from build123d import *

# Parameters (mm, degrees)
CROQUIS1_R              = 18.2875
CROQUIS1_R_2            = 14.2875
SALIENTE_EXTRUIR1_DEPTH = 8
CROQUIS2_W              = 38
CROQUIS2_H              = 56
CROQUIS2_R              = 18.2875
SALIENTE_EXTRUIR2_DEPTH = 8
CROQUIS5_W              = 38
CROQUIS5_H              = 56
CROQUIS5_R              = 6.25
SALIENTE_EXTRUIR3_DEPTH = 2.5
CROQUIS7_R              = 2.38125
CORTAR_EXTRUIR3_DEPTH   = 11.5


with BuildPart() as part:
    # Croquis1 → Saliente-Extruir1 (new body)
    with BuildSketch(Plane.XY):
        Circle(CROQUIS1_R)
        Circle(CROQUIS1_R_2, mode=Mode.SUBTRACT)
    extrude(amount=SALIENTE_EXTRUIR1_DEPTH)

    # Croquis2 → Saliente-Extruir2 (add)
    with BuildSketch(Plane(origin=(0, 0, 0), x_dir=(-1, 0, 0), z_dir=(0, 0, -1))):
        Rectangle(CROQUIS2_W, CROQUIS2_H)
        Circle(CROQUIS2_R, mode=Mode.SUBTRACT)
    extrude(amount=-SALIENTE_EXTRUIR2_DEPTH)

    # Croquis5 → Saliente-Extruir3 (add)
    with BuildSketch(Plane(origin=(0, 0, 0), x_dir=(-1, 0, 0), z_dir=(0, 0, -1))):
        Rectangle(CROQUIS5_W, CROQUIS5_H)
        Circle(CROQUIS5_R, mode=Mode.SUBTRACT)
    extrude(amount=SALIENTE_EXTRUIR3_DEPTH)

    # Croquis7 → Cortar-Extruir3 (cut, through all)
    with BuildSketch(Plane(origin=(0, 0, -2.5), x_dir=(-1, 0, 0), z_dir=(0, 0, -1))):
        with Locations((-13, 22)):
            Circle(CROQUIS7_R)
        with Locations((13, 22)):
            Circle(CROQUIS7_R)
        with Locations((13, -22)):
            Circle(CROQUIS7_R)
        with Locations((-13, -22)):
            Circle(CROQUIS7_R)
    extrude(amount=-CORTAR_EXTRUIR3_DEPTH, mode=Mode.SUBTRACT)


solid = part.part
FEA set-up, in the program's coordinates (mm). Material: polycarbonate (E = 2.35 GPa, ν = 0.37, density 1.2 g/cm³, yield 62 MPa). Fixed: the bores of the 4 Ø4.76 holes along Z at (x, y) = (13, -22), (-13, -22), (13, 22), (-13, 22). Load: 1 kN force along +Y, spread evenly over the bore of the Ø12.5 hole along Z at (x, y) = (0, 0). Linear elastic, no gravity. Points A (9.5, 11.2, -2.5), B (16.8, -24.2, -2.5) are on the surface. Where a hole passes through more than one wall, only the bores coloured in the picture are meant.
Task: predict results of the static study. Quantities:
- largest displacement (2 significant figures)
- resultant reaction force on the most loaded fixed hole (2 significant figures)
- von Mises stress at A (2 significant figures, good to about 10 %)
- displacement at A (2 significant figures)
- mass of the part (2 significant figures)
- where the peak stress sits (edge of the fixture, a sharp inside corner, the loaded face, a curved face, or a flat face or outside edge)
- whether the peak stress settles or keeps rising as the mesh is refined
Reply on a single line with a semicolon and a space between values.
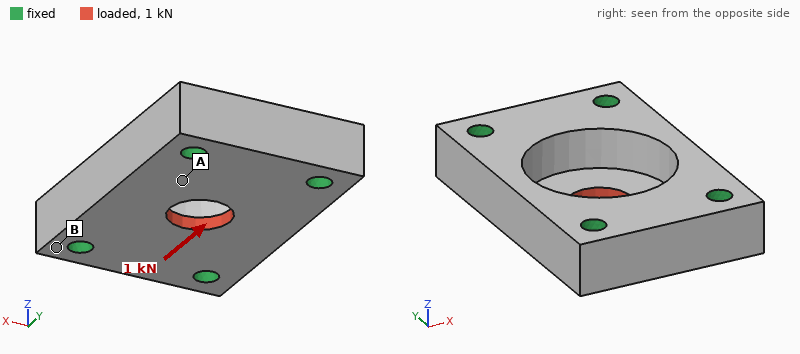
65 µm; 260 N; 6.0 MPa; 25 µm; 19 g; a sharp inside corner; keeps rising
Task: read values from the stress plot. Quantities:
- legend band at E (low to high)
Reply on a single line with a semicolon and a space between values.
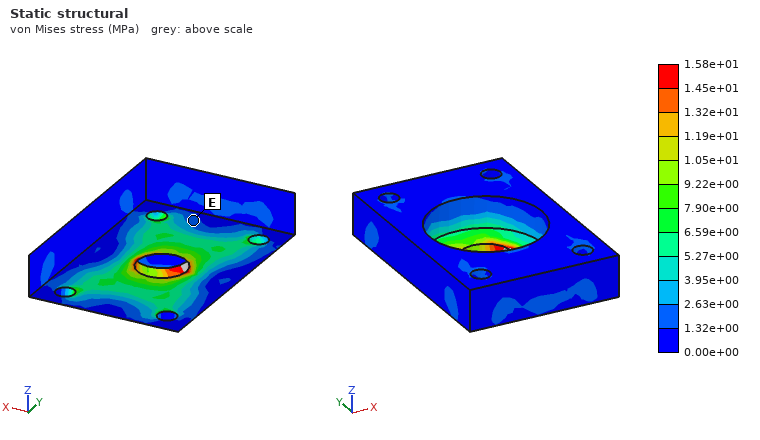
1.32e+00 to 2.63e+00 MPa
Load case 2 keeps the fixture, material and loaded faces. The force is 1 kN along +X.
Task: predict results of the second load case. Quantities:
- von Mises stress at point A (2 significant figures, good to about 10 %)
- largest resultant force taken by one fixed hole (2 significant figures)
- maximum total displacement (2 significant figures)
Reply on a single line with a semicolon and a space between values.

8.1 MPa; 300 N; 0.11 mm
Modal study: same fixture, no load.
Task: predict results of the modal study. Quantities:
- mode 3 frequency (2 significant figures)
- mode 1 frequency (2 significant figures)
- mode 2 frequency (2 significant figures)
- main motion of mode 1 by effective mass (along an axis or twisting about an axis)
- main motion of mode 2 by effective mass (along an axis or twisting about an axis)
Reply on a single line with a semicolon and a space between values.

8600 Hz; 6500 Hz; 7200 Hz; along Z; twisting about Y
